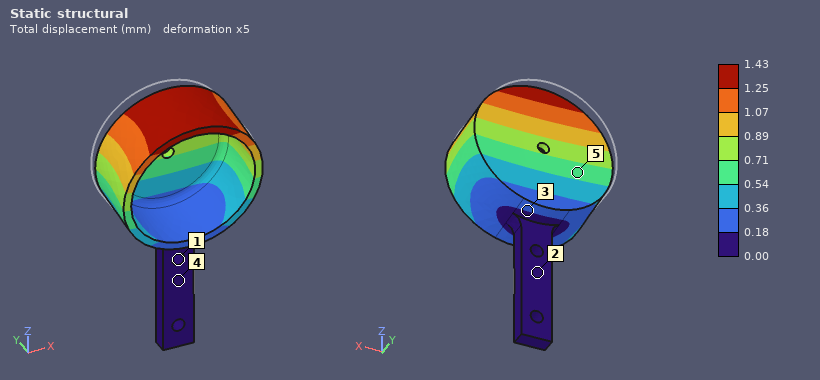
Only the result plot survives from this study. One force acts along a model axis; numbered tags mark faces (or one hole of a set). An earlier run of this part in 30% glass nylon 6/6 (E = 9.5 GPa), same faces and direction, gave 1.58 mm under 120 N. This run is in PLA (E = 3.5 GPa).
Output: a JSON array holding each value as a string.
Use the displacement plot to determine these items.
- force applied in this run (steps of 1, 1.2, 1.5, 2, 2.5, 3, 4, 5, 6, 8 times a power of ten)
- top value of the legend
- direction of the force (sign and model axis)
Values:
["40 N", "1.43 mm", "-Y"]
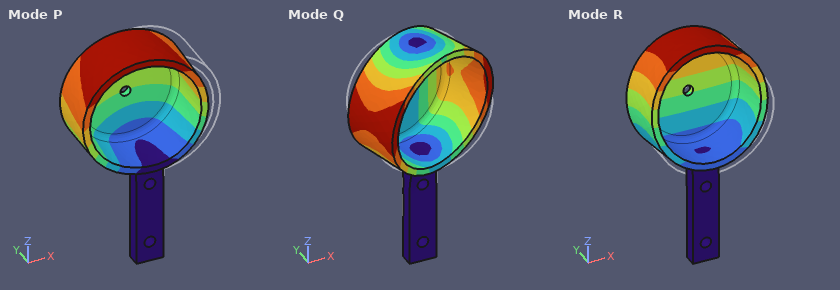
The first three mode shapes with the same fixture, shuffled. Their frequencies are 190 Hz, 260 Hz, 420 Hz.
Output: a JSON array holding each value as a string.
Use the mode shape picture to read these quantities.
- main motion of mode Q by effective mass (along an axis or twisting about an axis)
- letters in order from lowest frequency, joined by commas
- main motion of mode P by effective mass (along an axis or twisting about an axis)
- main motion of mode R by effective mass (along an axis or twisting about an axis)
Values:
["twisting about Z", "R, P, Q", "along X", "along Y"]
